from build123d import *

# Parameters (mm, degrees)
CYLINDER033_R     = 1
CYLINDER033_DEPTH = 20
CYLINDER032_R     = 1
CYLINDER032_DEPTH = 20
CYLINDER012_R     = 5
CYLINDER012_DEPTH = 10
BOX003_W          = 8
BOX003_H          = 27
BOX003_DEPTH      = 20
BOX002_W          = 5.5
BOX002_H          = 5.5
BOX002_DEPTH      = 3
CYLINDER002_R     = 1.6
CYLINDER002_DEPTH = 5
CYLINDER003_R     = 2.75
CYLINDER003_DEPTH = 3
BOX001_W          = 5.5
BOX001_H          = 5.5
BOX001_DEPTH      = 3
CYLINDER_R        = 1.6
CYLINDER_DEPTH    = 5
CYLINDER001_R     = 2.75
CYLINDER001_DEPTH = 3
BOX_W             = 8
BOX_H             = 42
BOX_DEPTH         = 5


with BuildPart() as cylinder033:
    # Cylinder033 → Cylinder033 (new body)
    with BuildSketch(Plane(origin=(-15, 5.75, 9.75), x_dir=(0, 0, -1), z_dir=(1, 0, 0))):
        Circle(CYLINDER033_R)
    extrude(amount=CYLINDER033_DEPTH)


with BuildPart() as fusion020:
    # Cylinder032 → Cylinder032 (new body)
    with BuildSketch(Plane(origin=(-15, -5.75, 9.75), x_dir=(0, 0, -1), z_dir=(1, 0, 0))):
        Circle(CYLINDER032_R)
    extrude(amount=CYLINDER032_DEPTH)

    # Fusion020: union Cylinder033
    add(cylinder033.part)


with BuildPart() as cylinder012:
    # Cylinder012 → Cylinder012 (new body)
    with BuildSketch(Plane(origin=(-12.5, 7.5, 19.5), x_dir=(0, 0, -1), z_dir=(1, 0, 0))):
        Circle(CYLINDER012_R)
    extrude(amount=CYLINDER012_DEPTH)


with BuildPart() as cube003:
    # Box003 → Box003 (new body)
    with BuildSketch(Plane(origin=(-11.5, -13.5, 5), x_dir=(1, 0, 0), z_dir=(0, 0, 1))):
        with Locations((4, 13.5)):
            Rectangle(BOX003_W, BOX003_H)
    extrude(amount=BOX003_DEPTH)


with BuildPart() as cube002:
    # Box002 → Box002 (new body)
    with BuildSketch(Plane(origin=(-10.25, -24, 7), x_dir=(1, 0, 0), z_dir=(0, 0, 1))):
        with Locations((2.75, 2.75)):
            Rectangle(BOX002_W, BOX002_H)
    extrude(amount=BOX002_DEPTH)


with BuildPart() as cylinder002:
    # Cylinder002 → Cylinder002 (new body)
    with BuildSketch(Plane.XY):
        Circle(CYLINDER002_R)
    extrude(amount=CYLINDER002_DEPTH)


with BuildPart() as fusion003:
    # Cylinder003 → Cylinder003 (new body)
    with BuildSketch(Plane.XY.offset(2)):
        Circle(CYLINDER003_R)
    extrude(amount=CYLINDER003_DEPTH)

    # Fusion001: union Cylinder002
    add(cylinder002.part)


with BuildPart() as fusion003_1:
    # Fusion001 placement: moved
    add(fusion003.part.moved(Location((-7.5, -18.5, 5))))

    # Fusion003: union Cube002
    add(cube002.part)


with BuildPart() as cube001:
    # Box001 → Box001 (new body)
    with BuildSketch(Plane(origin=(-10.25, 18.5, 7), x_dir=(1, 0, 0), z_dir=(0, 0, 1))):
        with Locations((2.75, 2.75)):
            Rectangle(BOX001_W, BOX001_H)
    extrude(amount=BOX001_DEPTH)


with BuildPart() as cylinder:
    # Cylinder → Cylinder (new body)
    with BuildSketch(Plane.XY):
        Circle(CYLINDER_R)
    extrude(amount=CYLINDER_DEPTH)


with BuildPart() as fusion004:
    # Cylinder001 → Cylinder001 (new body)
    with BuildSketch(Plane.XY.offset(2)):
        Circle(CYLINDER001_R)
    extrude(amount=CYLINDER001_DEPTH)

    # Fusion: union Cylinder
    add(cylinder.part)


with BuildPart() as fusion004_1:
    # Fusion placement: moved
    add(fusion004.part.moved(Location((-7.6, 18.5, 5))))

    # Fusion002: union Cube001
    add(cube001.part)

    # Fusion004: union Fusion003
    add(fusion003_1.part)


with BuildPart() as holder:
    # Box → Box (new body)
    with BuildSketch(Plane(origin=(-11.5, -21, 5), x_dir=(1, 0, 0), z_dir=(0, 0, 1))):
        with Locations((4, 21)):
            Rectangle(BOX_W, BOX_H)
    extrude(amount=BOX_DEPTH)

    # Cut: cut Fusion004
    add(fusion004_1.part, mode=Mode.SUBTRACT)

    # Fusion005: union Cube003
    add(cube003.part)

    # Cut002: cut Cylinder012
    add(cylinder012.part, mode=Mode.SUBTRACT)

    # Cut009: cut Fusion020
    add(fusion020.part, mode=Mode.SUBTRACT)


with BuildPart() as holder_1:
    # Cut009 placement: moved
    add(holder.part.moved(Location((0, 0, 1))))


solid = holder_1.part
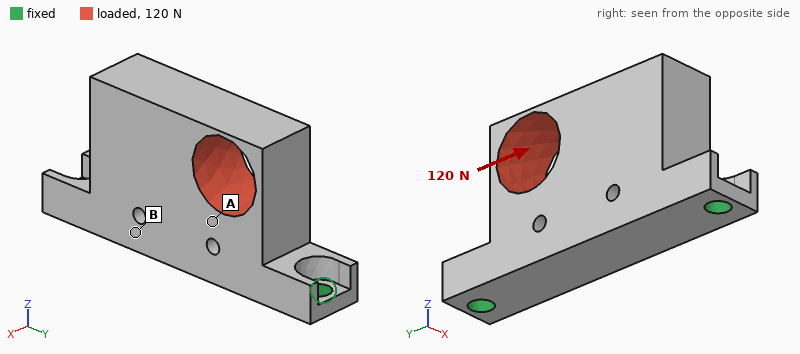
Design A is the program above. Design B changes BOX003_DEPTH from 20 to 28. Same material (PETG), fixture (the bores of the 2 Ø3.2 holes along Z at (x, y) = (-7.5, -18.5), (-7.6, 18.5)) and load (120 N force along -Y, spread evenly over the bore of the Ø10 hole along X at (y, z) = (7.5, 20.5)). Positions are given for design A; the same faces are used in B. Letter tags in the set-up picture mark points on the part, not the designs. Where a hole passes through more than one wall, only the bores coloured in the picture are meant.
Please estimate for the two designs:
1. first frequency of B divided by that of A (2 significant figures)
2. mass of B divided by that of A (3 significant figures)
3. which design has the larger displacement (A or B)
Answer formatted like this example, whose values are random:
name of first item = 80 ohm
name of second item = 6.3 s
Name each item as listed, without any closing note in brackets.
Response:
first frequency of B divided by that of A = 0.54
mass of B divided by that of A = 1.43
which design has the larger displacement = A
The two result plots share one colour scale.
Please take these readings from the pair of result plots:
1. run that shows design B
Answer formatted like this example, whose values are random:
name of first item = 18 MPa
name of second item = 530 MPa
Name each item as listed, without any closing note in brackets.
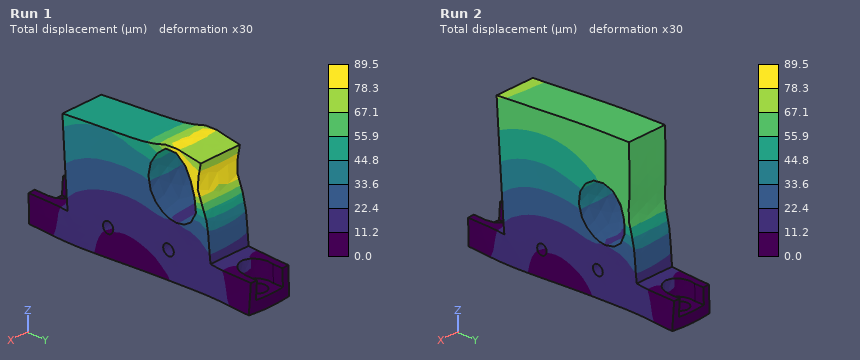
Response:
run that shows design B = Run 2
